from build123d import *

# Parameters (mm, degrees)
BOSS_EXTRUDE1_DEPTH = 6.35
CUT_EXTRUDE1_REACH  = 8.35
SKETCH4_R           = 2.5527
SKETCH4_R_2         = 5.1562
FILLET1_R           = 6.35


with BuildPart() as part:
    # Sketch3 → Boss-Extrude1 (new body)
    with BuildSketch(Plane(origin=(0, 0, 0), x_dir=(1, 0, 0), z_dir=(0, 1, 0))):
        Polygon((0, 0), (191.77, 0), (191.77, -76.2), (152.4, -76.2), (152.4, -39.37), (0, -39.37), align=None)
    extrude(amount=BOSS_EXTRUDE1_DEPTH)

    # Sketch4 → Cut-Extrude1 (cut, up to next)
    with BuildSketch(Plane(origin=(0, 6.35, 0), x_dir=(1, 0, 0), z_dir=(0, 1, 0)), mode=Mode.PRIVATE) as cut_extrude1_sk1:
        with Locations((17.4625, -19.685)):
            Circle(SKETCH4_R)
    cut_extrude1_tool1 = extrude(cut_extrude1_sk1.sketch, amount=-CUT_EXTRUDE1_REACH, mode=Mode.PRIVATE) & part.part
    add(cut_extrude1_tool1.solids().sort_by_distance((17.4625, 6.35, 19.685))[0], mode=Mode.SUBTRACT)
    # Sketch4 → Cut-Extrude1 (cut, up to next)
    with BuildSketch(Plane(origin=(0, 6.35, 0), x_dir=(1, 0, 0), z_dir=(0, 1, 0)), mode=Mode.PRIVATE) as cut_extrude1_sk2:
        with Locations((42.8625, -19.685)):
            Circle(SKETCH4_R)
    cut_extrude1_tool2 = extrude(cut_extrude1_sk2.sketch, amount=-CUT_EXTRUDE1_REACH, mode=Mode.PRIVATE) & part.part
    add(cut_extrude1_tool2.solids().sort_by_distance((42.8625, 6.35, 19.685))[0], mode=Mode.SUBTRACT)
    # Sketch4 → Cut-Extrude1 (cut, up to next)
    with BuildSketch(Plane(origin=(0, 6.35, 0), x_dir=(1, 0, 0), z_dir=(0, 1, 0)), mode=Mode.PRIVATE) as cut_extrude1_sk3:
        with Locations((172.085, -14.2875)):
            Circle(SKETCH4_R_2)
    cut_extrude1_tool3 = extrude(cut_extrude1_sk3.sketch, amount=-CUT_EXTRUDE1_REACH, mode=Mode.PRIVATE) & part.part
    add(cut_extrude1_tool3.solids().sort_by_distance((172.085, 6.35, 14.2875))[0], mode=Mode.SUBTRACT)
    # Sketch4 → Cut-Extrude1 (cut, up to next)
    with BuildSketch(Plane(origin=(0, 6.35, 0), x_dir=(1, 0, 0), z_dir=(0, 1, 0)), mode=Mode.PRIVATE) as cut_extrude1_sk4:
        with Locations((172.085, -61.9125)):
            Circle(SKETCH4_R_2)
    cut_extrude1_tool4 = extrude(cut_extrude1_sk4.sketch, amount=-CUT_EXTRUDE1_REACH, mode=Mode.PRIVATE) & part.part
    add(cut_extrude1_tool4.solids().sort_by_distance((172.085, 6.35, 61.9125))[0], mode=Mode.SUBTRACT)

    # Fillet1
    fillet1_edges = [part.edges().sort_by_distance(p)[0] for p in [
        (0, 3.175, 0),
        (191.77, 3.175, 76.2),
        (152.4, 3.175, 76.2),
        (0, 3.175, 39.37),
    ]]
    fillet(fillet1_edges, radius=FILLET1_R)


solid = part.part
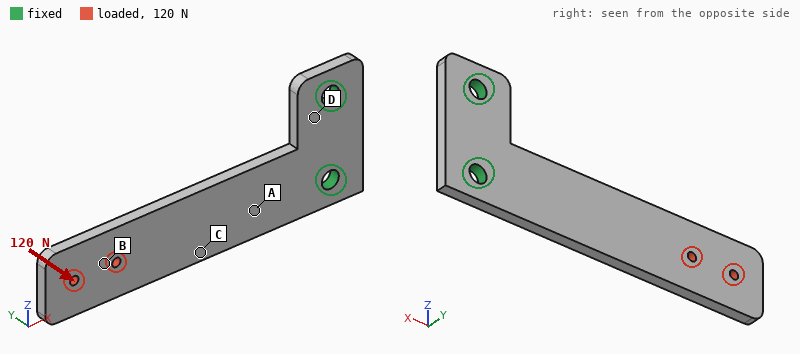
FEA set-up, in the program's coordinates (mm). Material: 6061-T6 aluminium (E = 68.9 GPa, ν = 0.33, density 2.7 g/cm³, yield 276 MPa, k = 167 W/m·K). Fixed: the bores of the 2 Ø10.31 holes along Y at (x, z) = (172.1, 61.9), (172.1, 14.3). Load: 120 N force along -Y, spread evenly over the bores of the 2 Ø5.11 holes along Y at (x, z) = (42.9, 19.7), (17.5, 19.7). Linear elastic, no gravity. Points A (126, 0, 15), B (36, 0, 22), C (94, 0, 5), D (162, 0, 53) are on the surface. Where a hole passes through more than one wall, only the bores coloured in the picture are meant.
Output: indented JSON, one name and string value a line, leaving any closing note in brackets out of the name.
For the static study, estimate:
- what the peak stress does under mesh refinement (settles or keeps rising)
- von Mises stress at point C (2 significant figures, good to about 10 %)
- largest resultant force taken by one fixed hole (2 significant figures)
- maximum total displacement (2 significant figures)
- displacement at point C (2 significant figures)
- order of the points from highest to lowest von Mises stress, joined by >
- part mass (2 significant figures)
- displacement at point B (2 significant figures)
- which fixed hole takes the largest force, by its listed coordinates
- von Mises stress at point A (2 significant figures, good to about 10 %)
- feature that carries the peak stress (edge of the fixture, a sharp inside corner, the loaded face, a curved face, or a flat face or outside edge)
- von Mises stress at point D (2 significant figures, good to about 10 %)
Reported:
{
  "what the peak stress does under mesh refinement": "keeps rising",
  "von Mises stress at point C": "29 MPa",
  "largest resultant force taken by one fixed hole": "150 N",
  "maximum total displacement": "2.4 mm",
  "displacement at point C": "0.64 mm",
  "order of the points from highest to lowest von Mises stress, joined by >": "A > C > D > B",
  "part mass": "150 g",
  "displacement at point B": "1.7 mm",
  "which fixed hole takes the largest force, by its listed coordinates": "(172.1, 14.3)",
  "von Mises stress at point A": "43 MPa",
  "feature that carries the peak stress": "edge of the fixture",
  "von Mises stress at point D": "16 MPa"
}
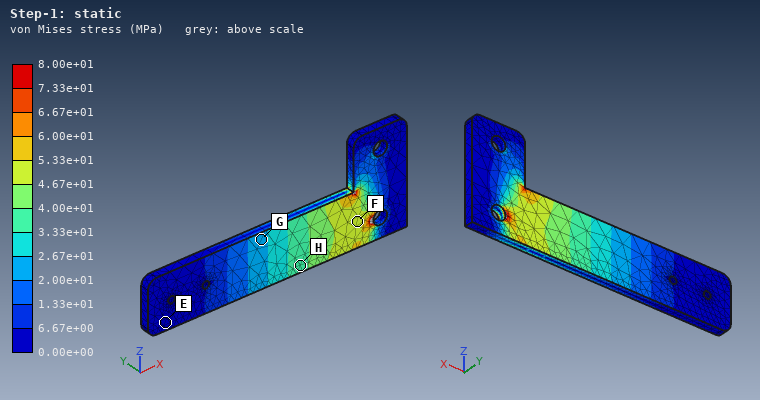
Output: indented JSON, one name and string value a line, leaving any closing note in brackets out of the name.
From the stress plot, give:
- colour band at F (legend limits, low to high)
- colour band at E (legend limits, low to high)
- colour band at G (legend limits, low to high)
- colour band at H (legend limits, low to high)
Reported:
{
  "colour band at F": "4.67e+01 to 5.33e+01 MPa",
  "colour band at E": "0.00e+00 to 6.67e+00 MPa",
  "colour band at G": "2.00e+01 to 2.67e+01 MPa",
  "colour band at H": "3.33e+01 to 4.00e+01 MPa"
}
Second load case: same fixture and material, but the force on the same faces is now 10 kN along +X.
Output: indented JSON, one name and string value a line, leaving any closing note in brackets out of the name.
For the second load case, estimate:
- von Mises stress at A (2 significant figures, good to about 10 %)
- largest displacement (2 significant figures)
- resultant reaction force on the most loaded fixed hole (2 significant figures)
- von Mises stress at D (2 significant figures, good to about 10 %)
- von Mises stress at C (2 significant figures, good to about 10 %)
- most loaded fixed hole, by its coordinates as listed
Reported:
{
  "von Mises stress at A": "40 MPa",
  "largest displacement": "91 µm",
  "resultant reaction force on the most loaded fixed hole": "8.7 kN",
  "von Mises stress at D": "12 MPa",
  "von Mises stress at C": "40 MPa",
  "most loaded fixed hole, by its coordinates as listed": "(172.1, 14.3)"
}
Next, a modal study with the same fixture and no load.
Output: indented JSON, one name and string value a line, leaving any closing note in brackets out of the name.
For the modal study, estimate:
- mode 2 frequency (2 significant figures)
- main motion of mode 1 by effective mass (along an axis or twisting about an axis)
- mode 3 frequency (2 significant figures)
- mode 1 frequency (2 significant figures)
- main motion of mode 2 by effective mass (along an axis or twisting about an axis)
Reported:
{
  "mode 2 frequency": "1100 Hz",
  "main motion of mode 1 by effective mass": "along Y",
  "mode 3 frequency": "1100 Hz",
  "mode 1 frequency": "190 Hz",
  "main motion of mode 2 by effective mass": "along Z"
}
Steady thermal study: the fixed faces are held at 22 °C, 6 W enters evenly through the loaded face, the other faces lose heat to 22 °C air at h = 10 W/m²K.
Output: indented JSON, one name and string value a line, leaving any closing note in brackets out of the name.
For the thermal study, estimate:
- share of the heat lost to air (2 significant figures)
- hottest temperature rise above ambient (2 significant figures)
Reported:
{
  "share of the heat lost to air": "24 %",
  "hottest temperature rise above ambient": "17 K"
}
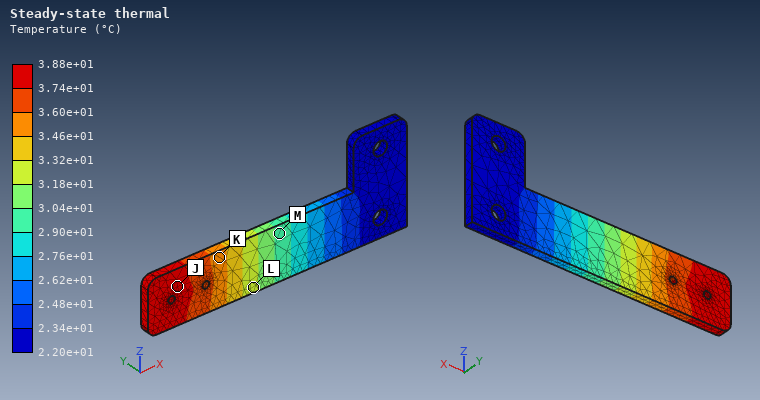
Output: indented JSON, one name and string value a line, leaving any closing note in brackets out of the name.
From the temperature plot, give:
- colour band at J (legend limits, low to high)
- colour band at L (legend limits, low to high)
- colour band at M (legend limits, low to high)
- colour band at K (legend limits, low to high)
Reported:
{
  "colour band at J": "3.74e+01 to 3.88e+01 °C",
  "colour band at L": "3.18e+01 to 3.32e+01 °C",
  "colour band at M": "2.90e+01 to 3.04e+01 °C",
  "colour band at K": "3.46e+01 to 3.60e+01 °C"
}
